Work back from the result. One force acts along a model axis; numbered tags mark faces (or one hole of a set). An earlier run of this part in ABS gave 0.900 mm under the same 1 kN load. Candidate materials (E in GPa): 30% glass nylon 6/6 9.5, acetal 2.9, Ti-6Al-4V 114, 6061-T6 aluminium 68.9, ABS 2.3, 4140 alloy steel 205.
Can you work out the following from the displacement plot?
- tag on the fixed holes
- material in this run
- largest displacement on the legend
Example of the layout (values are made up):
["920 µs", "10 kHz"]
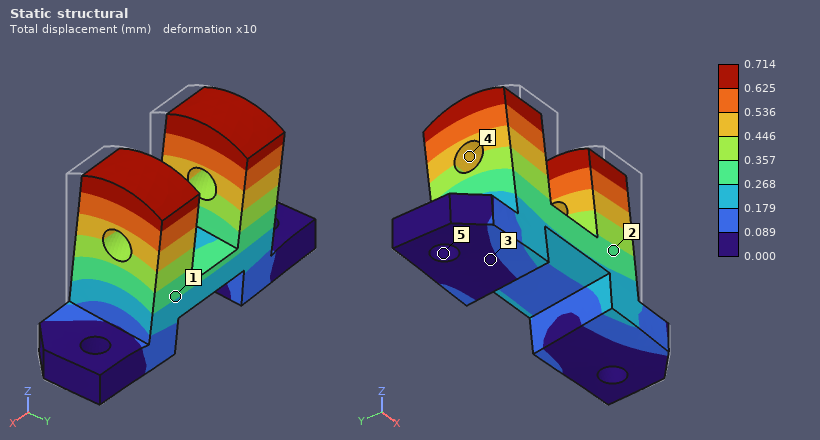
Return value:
["5", "acetal", "0.714 mm"]
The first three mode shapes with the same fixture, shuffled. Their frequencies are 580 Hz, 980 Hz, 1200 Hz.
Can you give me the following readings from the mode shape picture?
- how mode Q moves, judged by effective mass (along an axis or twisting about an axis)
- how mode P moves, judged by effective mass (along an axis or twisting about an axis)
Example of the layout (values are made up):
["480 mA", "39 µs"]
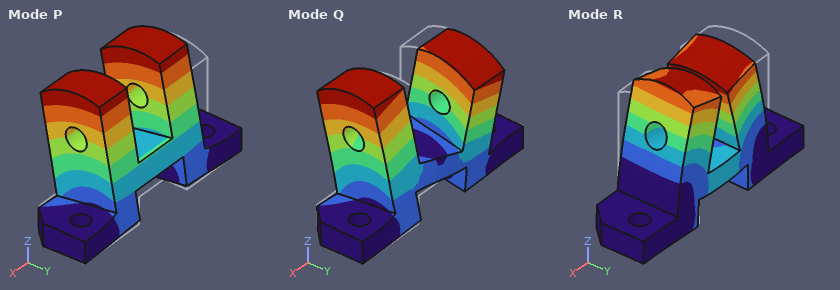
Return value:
["twisting about Z", "along Y"]
